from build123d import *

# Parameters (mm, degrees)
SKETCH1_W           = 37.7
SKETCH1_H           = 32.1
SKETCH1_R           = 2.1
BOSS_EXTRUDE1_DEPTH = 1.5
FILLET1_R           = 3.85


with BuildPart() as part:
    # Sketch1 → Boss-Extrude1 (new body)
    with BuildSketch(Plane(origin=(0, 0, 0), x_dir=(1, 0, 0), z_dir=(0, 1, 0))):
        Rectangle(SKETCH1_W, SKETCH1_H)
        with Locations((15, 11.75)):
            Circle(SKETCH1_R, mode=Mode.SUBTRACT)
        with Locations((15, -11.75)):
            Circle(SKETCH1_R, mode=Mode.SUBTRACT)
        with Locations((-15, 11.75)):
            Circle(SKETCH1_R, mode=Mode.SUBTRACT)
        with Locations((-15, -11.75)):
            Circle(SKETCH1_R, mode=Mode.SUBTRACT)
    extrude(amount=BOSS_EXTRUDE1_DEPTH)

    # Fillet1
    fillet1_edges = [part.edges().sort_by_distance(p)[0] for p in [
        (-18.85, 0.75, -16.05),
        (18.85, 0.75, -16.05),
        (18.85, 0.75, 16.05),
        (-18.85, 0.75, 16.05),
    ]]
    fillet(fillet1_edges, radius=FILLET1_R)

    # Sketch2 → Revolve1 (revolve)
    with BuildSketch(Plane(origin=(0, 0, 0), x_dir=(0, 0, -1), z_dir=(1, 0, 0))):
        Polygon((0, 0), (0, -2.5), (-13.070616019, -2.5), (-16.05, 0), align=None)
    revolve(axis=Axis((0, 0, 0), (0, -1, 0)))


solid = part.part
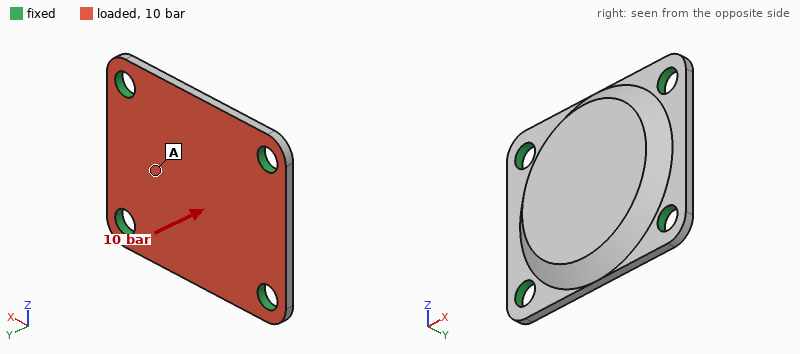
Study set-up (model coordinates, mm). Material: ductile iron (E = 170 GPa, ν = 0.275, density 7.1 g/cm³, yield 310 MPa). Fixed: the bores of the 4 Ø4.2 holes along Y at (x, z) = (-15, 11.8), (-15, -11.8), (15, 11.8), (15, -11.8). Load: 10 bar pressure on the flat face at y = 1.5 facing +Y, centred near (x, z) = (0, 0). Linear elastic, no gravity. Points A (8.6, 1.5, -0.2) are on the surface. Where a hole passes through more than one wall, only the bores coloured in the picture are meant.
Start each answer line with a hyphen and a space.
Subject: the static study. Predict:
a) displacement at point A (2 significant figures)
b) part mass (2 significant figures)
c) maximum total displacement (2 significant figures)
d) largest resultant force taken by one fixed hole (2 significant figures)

- 5.4 µm
- 24 g
- 7.0 µm
- 390 N
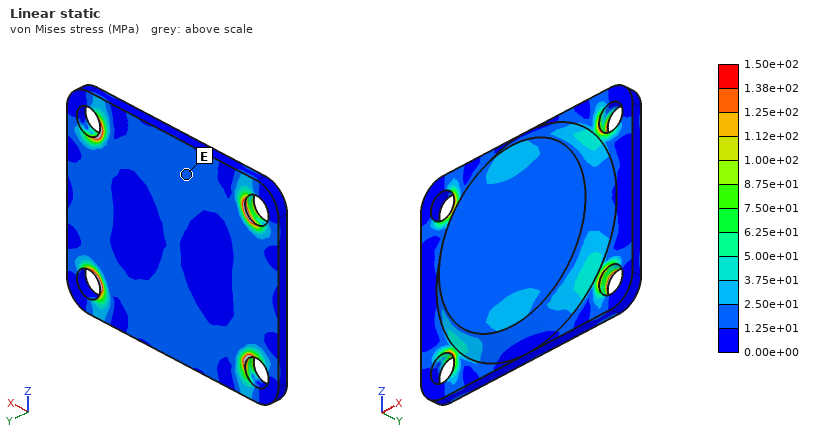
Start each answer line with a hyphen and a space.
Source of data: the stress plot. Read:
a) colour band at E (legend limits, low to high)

- 1.25e+01 to 2.50e+01 MPa
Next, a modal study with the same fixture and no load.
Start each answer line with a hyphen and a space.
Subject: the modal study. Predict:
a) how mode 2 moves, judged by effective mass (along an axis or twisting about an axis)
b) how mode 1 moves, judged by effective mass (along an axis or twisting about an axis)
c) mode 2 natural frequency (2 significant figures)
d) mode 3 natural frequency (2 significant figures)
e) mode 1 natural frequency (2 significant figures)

- twisting about X
- along Y
- 18 kHz
- 24 kHz
- 13 kHz
